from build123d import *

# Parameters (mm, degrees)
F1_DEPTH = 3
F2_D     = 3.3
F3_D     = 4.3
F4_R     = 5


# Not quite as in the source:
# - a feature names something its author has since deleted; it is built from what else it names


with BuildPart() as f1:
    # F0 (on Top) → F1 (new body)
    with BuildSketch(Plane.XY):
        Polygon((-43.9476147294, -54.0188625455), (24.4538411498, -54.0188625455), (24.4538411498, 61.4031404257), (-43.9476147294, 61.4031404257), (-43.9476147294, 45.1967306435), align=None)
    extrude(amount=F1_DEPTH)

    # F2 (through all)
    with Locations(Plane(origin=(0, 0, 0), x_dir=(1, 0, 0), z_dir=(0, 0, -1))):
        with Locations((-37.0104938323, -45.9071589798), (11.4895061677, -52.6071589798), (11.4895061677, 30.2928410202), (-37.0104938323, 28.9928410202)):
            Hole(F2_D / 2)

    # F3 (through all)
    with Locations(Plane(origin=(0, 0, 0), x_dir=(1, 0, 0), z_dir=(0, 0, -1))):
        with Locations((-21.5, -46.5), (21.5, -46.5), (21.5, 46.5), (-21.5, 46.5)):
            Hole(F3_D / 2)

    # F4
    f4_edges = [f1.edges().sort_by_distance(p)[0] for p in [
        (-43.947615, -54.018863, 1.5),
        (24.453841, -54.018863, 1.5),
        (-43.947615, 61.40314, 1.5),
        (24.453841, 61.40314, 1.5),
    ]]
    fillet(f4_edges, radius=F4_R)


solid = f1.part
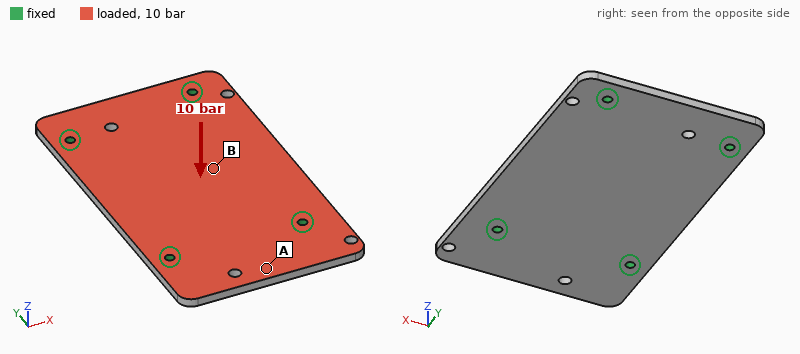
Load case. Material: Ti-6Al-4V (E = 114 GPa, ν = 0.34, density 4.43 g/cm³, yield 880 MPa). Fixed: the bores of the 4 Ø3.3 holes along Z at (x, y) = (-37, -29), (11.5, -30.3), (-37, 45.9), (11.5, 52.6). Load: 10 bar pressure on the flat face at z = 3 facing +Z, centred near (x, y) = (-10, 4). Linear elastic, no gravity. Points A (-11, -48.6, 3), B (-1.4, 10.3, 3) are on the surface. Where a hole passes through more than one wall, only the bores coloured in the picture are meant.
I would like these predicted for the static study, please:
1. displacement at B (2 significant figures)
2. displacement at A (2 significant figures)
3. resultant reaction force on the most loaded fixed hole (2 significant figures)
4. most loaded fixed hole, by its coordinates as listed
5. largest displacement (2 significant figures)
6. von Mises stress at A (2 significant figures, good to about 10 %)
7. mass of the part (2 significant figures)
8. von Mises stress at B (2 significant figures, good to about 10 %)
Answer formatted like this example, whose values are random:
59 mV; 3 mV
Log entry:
0.53 mm; 0.13 mm; 2.4 kN; (11.5, -30.3); 0.59 mm; 58 MPa; 100 g; 170 MPa
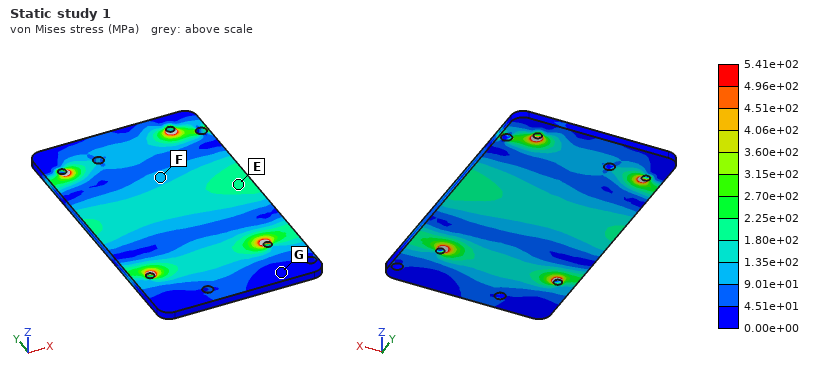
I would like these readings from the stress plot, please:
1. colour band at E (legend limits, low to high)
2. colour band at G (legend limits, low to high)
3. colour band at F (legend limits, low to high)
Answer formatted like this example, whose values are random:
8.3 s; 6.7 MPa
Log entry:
1.80e+02 to 2.25e+02 MPa; 0.00e+00 to 4.51e+01 MPa; 9.01e+01 to 1.35e+02 MPa
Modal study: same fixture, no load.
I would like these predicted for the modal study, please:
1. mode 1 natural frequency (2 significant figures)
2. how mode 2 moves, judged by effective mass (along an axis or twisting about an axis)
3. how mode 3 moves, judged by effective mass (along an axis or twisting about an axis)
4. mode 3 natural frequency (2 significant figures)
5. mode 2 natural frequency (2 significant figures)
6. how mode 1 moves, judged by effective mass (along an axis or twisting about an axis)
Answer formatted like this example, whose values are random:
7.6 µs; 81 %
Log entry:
2100 Hz; twisting about Y; along Z; 3300 Hz; 3100 Hz; along Z
